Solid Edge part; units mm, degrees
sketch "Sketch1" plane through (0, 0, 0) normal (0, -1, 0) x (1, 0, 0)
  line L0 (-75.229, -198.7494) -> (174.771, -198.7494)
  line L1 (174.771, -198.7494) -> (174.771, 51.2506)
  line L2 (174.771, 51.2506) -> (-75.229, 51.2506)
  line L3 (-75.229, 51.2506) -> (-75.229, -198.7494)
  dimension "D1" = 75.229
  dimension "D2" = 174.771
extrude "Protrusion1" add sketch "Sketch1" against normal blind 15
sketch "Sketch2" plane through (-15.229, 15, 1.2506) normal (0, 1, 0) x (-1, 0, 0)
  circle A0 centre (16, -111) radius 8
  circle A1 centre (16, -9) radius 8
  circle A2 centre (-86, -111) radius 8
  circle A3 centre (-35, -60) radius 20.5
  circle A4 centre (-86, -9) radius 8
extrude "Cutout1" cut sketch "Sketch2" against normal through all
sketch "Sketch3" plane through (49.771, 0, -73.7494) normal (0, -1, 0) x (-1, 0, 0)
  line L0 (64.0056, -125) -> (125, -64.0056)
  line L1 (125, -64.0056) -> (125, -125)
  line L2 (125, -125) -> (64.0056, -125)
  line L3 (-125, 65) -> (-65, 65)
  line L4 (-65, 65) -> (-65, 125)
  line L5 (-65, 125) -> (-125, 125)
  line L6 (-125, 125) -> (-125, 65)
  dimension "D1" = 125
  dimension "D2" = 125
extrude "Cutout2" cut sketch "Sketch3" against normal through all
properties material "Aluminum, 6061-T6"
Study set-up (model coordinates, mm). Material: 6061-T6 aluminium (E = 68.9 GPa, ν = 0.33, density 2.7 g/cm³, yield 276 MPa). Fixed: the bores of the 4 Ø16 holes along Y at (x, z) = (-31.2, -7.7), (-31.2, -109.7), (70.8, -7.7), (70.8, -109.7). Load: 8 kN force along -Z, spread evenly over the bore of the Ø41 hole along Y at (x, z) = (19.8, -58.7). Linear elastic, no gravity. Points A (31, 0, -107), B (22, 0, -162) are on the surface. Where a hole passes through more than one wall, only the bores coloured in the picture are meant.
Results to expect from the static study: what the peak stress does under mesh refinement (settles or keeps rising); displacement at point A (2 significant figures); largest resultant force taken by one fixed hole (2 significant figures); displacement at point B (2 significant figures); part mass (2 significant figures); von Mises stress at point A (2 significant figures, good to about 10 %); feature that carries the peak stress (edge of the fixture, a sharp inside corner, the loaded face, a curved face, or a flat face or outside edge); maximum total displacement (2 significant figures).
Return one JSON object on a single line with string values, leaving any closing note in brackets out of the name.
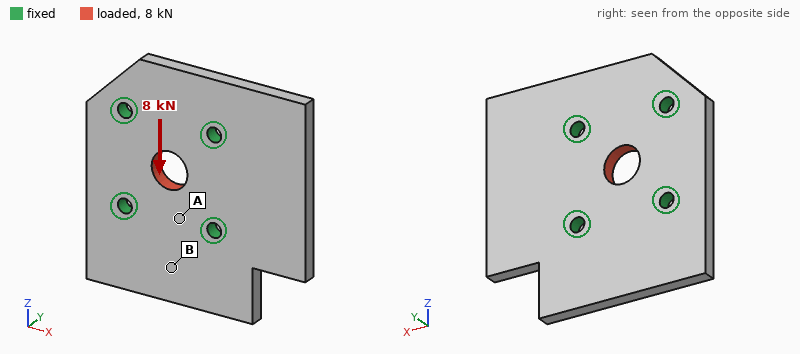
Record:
{"what the peak stress does under mesh refinement": "keeps rising", "displacement at point A": "1.9 µm", "largest resultant force taken by one fixed hole": "2.1 kN", "displacement at point B": "1.1 µm", "part mass": "2.2 kg", "von Mises stress at point A": "2.1 MPa", "feature that carries the peak stress": "edge of the fixture", "maximum total displacement": "3.4 µm"}
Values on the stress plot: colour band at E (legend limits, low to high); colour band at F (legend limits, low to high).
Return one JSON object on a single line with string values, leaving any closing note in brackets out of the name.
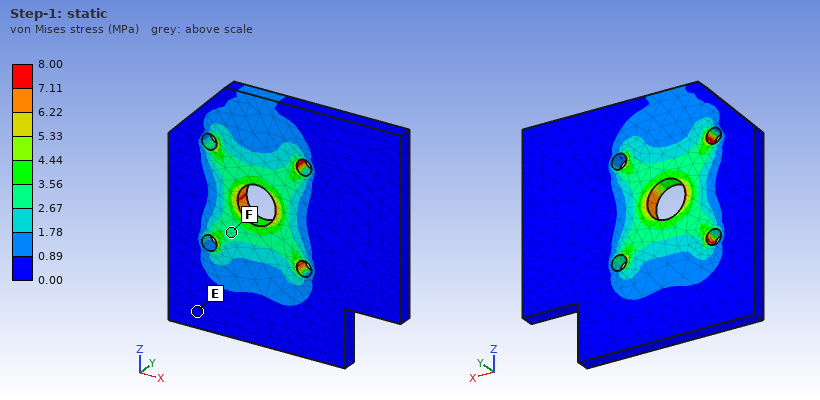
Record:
{"colour band at E": "0.00 to 0.89 MPa", "colour band at F": "2.67 to 3.56 MPa"}
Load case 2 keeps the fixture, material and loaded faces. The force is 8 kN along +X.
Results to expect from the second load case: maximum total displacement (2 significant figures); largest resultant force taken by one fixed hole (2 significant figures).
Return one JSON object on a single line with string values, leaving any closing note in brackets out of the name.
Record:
{"maximum total displacement": "3.6 µm", "largest resultant force taken by one fixed hole": "2.1 kN"}
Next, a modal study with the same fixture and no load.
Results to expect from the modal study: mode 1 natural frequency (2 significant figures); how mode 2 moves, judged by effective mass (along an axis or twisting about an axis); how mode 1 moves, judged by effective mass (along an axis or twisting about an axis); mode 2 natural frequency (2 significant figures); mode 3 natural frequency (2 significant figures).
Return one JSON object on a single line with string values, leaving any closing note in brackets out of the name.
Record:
{"mode 1 natural frequency": "1100 Hz", "how mode 2 moves, judged by effective mass": "along Y", "how mode 1 moves, judged by effective mass": "along Y", "mode 2 natural frequency": "1500 Hz", "mode 3 natural frequency": "1700 Hz"}
